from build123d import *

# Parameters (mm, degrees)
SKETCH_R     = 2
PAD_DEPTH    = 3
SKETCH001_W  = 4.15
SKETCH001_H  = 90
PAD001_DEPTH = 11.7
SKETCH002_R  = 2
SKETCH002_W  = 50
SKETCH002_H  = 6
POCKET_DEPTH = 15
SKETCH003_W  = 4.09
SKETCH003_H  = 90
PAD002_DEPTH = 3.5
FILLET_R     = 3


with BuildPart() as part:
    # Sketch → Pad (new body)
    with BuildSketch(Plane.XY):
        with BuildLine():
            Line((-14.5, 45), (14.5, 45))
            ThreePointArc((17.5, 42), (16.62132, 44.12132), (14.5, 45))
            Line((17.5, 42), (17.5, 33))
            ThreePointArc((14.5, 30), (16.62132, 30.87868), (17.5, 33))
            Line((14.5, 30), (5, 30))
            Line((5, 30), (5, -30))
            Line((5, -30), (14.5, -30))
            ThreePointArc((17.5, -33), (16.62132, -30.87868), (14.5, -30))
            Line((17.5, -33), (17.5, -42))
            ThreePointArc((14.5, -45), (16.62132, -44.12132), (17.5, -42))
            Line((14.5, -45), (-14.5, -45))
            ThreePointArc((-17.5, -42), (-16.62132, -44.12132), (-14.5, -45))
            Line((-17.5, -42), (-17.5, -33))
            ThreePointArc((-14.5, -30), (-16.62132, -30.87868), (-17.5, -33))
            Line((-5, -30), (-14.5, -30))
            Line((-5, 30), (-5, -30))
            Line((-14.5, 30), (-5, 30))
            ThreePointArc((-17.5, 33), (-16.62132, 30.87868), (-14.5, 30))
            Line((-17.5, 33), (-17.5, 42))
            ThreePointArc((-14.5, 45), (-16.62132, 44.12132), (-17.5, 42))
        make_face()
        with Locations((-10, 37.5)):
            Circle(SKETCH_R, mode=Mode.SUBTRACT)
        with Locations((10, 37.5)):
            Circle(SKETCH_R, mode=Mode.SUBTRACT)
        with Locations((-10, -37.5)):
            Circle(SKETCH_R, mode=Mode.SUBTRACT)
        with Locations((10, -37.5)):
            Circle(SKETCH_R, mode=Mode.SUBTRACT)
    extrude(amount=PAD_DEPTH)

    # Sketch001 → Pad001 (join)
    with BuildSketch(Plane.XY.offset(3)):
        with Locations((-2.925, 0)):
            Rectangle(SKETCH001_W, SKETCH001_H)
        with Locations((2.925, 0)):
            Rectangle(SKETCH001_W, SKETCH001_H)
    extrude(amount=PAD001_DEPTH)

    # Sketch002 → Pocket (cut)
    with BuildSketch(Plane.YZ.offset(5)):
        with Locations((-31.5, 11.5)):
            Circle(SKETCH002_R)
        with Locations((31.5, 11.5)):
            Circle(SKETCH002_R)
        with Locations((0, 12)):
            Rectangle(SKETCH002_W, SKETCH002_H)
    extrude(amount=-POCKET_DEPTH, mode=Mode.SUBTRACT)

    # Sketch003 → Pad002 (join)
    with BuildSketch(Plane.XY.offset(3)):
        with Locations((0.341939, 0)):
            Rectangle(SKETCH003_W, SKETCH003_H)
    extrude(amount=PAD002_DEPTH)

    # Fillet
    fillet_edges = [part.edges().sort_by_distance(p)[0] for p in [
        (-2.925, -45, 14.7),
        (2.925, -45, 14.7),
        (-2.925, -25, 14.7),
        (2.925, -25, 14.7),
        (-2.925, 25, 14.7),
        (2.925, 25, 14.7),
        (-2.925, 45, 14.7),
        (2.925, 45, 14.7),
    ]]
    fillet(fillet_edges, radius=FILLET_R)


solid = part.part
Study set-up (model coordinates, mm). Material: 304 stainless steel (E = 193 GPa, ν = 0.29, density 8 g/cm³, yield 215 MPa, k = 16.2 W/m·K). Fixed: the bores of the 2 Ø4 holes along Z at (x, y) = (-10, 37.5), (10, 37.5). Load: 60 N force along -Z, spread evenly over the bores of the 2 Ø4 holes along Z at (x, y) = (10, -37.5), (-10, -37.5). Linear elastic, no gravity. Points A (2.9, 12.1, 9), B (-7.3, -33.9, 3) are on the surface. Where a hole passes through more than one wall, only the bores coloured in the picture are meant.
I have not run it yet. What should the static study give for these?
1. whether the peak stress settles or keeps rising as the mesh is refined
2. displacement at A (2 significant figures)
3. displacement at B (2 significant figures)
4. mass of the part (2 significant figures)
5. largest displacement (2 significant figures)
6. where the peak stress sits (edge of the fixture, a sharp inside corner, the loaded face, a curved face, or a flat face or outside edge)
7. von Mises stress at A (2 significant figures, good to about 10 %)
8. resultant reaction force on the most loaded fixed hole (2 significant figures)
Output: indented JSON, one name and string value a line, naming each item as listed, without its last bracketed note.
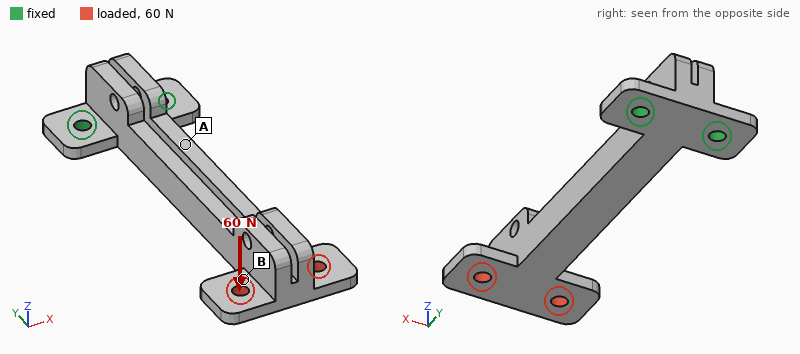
{
  "whether the peak stress settles or keeps rising as the mesh is refined": "keeps rising",
  "displacement at A": "0.030 mm",
  "displacement at B": "0.12 mm",
  "mass of the part": "91 g",
  "largest displacement": "0.14 mm",
  "where the peak stress sits": "edge of the fixture",
  "von Mises stress at A": "25 MPa",
  "resultant reaction force on the most loaded fixed hole": "64 N"
}
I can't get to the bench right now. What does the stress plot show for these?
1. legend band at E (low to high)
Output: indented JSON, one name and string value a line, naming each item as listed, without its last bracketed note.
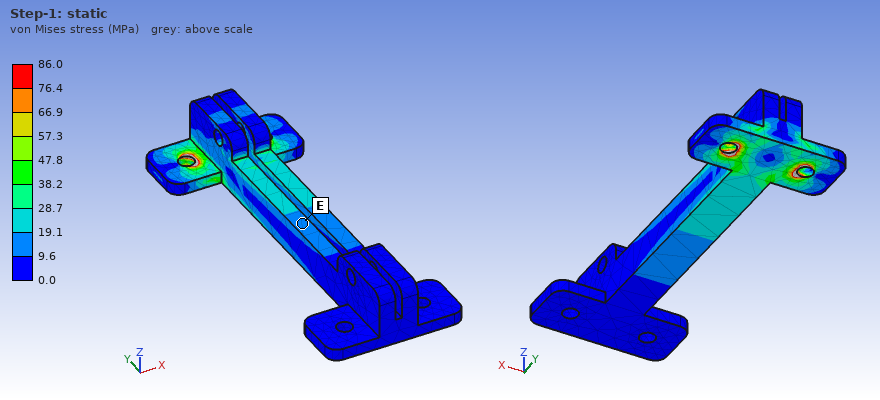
{
  "legend band at E": "9.6 to 19.1 MPa"
}
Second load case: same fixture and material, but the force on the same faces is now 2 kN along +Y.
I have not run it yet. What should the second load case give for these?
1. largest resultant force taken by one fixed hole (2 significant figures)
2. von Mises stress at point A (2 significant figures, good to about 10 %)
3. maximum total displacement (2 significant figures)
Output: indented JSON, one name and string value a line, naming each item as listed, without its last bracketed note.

{
  "largest resultant force taken by one fixed hole": "1.0 kN",
  "von Mises stress at point A": "24 MPa",
  "maximum total displacement": "0.15 mm"
}
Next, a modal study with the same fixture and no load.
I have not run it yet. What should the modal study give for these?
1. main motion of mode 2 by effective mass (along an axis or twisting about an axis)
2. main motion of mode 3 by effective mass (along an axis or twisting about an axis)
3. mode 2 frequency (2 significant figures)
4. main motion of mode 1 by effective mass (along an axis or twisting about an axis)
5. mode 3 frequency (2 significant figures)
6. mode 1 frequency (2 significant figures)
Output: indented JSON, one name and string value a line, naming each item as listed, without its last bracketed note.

{
  "main motion of mode 2 by effective mass": "along X",
  "main motion of mode 3 by effective mass": "twisting about Y",
  "mode 2 frequency": "920 Hz",
  "main motion of mode 1 by effective mass": "along Z",
  "mode 3 frequency": "3200 Hz",
  "mode 1 frequency": "590 Hz"
}
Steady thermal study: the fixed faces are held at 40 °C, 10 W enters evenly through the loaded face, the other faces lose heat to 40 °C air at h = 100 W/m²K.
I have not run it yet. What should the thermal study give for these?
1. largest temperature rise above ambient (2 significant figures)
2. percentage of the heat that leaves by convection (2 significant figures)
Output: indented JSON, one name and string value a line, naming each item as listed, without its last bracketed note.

{
  "largest temperature rise above ambient": "70 K",
  "percentage of the heat that leaves by convection": "99 %"
}
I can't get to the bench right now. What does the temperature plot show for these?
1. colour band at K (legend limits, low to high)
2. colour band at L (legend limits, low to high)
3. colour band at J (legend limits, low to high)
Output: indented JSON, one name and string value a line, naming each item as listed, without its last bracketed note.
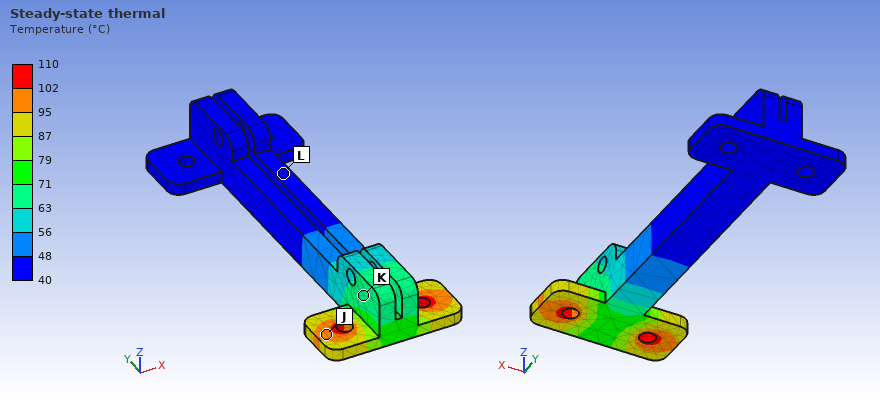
{
  "colour band at K": "63 to 71 °C",
  "colour band at L": "40 to 48 °C",
  "colour band at J": "95 to 102 °C"
}
